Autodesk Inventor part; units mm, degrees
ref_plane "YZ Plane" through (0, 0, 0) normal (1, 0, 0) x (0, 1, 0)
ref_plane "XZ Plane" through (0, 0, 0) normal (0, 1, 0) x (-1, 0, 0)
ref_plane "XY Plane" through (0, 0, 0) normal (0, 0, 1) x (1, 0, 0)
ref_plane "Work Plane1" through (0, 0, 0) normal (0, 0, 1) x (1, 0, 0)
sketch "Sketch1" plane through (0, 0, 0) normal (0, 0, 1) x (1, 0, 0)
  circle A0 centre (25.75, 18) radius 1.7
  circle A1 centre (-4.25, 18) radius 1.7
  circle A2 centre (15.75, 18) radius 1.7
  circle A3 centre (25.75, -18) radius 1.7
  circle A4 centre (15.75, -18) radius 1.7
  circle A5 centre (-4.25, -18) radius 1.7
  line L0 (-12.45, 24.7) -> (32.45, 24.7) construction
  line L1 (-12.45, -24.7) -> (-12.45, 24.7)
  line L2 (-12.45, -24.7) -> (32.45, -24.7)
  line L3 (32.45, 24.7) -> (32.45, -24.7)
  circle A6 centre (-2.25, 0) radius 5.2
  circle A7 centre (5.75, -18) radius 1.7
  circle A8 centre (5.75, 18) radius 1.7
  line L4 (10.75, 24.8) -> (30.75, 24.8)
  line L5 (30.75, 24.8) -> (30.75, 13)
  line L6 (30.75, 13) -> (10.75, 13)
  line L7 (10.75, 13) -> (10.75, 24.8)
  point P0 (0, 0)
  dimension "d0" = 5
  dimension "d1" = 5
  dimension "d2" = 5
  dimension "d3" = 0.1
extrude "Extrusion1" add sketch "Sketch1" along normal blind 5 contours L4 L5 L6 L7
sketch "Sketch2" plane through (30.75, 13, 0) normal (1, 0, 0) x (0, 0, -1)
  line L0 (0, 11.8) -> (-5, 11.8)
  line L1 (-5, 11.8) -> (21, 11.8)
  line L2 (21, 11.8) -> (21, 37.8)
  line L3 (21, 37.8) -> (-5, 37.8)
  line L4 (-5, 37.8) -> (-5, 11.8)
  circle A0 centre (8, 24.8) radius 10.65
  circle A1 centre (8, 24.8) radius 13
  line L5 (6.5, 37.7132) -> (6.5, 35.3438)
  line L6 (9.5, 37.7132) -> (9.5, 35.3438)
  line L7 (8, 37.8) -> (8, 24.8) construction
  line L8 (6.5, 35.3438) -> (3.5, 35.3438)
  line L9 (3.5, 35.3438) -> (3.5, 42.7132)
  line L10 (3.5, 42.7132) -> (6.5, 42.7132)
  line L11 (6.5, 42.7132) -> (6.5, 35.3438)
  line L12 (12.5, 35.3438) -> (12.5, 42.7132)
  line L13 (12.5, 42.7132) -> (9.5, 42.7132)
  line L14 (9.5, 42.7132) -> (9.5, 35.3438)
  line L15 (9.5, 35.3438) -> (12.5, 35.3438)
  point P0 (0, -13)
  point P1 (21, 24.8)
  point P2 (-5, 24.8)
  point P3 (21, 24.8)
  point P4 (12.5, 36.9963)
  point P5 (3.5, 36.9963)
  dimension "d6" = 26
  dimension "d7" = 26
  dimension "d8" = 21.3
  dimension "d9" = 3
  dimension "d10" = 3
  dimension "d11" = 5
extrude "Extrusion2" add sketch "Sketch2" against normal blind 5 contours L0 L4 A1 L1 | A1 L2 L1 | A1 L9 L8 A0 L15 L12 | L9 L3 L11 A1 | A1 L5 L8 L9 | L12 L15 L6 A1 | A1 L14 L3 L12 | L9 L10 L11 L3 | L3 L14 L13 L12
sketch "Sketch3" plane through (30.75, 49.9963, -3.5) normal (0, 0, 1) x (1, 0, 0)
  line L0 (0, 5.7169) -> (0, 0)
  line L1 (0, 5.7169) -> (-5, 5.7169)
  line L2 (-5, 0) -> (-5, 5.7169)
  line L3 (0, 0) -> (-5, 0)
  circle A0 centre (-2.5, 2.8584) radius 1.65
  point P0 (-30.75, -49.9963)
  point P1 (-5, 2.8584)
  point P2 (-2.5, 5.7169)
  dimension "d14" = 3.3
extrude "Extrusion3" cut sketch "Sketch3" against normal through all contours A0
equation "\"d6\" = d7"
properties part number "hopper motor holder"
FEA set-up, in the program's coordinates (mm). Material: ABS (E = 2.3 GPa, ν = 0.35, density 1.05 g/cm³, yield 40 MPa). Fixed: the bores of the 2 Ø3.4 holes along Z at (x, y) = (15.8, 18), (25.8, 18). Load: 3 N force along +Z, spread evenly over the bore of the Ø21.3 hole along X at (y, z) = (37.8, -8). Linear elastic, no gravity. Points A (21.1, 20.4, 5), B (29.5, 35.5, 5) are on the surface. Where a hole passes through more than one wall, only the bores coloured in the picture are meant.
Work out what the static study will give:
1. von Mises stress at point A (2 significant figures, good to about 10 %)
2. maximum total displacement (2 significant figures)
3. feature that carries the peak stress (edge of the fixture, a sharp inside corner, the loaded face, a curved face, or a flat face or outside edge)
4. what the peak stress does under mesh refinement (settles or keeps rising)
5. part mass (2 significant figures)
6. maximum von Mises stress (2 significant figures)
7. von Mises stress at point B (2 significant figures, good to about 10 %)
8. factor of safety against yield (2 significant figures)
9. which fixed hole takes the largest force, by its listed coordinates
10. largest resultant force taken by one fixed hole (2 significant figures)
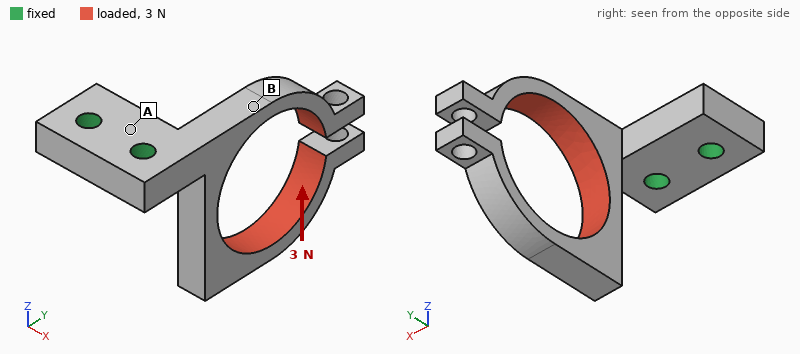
0.38 MPa
0.49 mm
the loaded face
settles
2.5 g
3.9 MPa
1.1 MPa
10
(25.8, 18)
3.2 N
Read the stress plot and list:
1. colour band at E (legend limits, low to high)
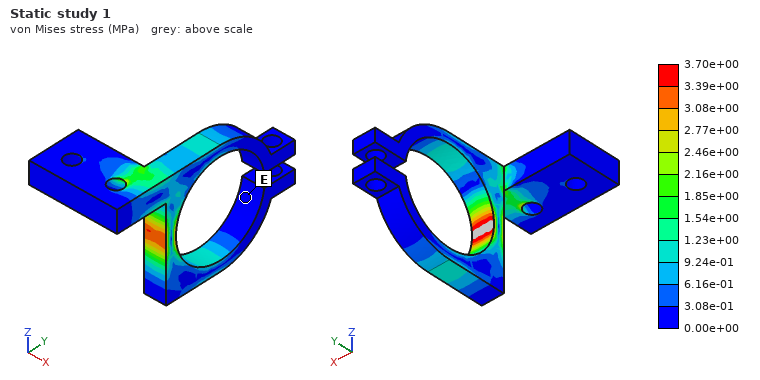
0.00e+00 to 3.08e-01 MPa
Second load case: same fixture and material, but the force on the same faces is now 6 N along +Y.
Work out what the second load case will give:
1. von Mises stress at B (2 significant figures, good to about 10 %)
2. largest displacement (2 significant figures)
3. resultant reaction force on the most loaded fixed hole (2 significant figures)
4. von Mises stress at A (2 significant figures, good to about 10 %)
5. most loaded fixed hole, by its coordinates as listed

0.99 MPa
0.49 mm
6.6 N
0.45 MPa
(25.8, 18)
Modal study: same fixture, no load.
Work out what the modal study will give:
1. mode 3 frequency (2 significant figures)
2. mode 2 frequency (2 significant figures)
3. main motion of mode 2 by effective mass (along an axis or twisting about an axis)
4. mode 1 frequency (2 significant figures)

790 Hz
460 Hz
along X
400 Hz
